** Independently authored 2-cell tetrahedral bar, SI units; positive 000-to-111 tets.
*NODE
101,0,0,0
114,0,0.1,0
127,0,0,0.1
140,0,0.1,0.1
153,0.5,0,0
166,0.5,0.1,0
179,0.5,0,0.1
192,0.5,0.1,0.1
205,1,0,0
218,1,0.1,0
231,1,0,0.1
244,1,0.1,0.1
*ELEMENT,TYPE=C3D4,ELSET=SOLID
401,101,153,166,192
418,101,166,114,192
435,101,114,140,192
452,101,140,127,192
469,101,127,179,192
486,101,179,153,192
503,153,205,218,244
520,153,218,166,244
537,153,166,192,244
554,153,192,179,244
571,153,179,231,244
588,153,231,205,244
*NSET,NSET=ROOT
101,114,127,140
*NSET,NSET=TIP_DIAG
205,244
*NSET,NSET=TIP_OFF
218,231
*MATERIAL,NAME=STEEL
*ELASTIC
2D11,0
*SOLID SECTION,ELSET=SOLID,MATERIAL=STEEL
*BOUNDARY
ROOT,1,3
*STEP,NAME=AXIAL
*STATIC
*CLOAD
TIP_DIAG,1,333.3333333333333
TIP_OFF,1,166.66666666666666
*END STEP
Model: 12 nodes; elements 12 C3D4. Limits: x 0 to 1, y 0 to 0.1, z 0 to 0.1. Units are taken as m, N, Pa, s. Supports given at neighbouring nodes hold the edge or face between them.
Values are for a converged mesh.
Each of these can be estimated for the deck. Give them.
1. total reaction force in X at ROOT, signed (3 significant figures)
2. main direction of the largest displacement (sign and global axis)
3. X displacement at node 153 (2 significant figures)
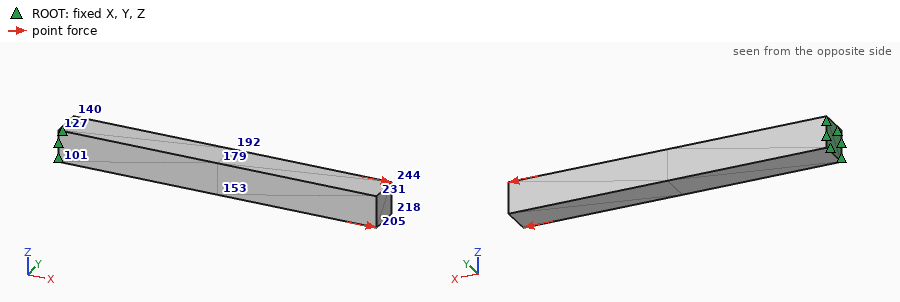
-1000 N
+X
2.5e-07 m
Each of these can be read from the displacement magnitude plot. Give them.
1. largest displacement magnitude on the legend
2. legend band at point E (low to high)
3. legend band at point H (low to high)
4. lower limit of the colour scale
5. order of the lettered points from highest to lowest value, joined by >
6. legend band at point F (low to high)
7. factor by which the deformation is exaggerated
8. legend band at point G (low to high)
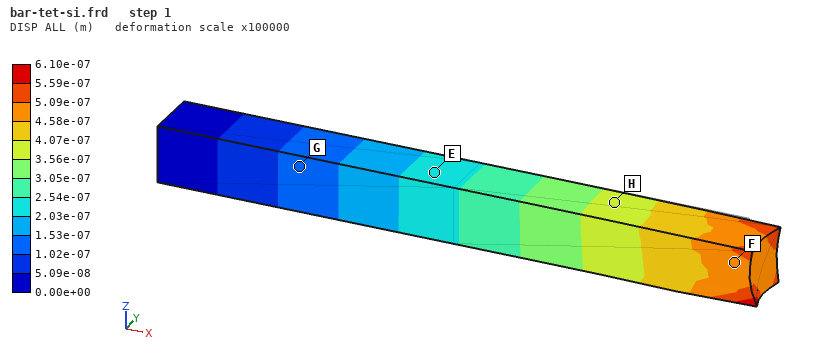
6.10e-07 m
2.03e-07 to 2.54e-07 m
3.56e-07 to 4.07e-07 m
0.00e+00 m
F > H > E > G
4.58e-07 to 5.09e-07 m
100000
1.02e-07 to 1.53e-07 m
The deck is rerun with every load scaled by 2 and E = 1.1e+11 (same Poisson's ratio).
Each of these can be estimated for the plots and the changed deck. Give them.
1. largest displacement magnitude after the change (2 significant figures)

2.2e-06 m
